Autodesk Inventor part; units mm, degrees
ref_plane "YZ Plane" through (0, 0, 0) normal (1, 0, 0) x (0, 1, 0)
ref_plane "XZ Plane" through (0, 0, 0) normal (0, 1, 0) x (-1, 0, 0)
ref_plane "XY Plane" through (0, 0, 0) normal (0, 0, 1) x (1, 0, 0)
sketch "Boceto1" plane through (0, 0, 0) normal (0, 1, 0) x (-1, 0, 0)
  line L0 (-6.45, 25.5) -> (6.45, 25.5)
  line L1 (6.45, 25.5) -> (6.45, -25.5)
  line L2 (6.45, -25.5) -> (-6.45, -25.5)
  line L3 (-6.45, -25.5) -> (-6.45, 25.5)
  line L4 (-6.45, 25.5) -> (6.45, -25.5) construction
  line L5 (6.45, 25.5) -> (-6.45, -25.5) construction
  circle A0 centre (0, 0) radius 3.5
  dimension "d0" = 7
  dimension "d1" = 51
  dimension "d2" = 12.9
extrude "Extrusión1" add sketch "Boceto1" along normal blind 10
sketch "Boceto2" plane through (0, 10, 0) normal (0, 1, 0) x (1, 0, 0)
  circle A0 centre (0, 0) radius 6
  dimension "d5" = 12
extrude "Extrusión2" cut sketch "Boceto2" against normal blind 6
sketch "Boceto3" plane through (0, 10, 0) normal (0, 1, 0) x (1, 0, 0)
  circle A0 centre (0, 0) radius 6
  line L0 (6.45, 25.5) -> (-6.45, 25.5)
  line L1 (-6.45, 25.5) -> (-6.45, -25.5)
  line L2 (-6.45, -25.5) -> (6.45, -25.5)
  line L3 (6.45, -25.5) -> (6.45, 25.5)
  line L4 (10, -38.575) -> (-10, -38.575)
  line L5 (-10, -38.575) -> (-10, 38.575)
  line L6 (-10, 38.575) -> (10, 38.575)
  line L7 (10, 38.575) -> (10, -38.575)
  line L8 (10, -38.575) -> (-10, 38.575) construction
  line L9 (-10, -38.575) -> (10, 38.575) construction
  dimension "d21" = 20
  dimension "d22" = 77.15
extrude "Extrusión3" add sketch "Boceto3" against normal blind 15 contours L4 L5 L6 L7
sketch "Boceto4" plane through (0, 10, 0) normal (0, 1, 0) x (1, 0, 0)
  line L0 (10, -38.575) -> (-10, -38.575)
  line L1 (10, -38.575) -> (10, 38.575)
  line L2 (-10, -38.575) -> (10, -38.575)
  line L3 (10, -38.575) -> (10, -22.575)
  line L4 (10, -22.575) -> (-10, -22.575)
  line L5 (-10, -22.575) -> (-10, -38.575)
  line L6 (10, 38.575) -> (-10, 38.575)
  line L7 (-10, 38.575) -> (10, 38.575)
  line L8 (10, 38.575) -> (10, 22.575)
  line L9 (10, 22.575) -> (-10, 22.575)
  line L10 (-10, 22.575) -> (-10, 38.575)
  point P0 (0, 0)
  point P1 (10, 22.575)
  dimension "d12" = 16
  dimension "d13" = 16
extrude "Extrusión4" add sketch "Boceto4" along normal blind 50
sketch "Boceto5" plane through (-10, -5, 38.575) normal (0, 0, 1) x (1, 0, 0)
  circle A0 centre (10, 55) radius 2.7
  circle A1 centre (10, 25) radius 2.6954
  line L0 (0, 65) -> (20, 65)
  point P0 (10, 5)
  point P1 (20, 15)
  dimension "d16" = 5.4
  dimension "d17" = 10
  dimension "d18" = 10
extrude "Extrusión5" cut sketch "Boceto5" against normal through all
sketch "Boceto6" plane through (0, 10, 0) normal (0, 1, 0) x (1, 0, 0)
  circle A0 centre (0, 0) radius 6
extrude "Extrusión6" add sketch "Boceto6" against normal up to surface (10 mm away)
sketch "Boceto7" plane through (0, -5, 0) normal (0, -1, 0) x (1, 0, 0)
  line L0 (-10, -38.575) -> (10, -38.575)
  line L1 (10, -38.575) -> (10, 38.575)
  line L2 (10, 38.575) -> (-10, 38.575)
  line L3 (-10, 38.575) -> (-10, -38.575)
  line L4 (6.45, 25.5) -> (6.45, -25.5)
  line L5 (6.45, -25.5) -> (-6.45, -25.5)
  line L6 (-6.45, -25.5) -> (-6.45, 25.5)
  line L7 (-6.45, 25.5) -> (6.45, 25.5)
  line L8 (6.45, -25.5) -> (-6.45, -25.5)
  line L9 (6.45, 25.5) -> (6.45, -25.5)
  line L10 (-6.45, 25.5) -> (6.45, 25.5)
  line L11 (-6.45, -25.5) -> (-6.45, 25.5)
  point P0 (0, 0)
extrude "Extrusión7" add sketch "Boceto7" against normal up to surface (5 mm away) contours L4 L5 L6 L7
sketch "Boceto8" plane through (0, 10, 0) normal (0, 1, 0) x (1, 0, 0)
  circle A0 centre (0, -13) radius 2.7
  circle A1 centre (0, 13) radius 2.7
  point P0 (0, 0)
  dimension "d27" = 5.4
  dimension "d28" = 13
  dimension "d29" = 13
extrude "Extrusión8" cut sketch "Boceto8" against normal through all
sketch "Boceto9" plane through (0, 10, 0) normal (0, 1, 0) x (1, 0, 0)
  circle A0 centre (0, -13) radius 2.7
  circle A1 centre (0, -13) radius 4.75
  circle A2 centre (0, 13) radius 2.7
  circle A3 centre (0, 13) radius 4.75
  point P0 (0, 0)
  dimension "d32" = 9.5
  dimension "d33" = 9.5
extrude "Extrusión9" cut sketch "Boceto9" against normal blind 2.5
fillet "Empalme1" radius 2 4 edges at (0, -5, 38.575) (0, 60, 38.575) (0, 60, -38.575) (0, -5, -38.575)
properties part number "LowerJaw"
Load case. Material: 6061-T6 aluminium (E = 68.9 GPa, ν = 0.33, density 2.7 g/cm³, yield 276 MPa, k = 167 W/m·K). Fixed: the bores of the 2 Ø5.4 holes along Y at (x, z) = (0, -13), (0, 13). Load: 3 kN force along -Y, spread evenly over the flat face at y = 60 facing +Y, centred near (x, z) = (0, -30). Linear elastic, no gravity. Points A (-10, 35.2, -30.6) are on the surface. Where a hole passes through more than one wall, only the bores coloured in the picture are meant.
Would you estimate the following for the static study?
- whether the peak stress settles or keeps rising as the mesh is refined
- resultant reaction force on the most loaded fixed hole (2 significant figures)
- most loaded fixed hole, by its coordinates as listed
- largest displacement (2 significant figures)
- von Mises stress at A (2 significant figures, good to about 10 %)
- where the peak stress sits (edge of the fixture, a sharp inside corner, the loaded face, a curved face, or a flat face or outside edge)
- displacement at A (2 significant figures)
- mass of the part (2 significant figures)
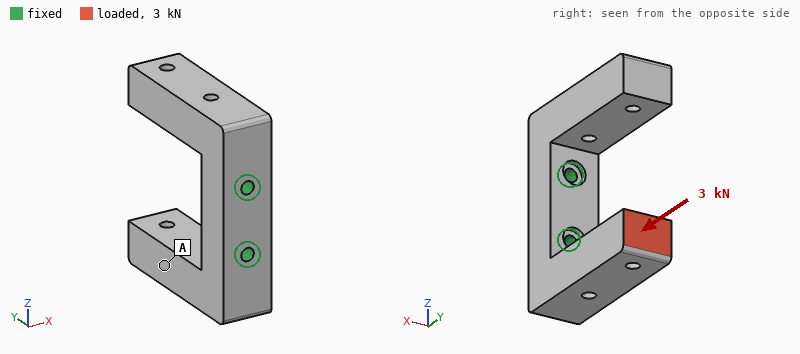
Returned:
keeps rising
3.5 kN
(0, -13)
91 µm
10 MPa
edge of the fixture
57 µm
140 g
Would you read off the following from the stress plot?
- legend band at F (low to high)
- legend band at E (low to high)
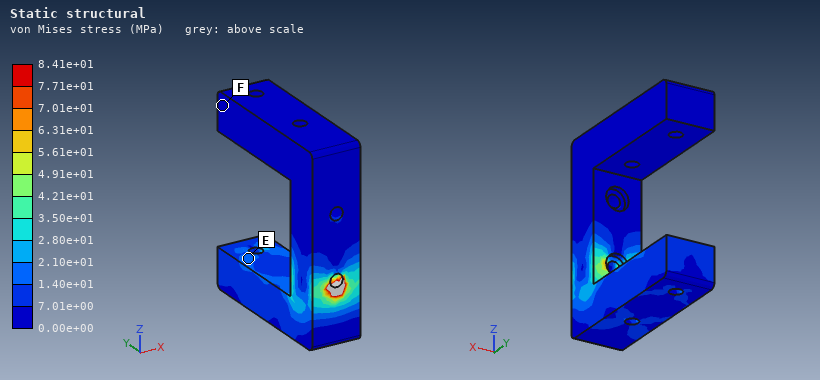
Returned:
0.00e+00 to 7.01e+00 MPa
1.40e+01 to 2.10e+01 MPa
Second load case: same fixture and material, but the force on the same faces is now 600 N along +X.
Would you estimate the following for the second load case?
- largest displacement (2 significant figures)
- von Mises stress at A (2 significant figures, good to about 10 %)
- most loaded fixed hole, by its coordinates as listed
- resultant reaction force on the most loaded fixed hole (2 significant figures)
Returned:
0.15 mm
14 MPa
(0, -13)
810 N
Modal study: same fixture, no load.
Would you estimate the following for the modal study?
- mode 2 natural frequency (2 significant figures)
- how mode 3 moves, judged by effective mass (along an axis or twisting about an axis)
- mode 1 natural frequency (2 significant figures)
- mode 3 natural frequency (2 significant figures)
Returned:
2500 Hz
along X
2400 Hz
2600 Hz
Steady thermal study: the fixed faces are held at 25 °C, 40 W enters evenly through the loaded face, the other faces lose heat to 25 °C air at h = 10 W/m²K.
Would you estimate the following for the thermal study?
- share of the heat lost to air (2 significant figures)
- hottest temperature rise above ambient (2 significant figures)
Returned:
3.9 %
56 K
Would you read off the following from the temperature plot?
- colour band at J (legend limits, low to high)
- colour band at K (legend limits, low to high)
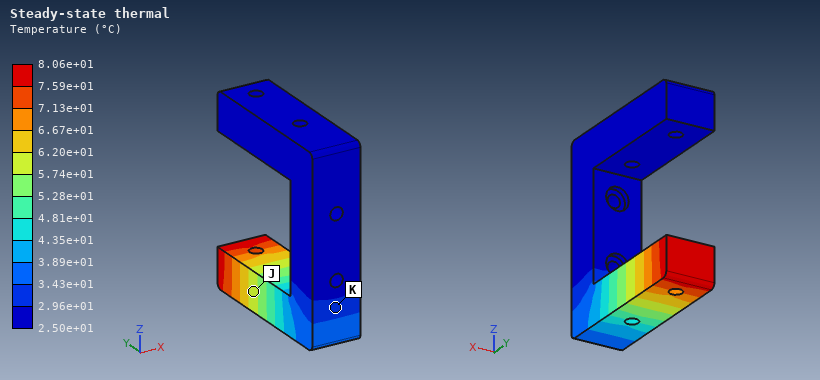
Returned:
5.74e+01 to 6.20e+01 °C
2.96e+01 to 3.43e+01 °C
